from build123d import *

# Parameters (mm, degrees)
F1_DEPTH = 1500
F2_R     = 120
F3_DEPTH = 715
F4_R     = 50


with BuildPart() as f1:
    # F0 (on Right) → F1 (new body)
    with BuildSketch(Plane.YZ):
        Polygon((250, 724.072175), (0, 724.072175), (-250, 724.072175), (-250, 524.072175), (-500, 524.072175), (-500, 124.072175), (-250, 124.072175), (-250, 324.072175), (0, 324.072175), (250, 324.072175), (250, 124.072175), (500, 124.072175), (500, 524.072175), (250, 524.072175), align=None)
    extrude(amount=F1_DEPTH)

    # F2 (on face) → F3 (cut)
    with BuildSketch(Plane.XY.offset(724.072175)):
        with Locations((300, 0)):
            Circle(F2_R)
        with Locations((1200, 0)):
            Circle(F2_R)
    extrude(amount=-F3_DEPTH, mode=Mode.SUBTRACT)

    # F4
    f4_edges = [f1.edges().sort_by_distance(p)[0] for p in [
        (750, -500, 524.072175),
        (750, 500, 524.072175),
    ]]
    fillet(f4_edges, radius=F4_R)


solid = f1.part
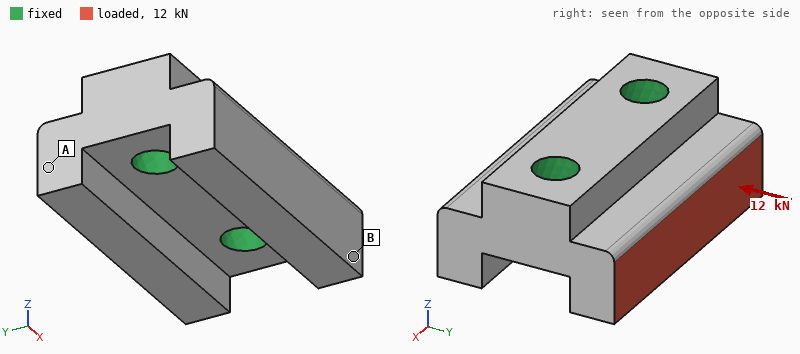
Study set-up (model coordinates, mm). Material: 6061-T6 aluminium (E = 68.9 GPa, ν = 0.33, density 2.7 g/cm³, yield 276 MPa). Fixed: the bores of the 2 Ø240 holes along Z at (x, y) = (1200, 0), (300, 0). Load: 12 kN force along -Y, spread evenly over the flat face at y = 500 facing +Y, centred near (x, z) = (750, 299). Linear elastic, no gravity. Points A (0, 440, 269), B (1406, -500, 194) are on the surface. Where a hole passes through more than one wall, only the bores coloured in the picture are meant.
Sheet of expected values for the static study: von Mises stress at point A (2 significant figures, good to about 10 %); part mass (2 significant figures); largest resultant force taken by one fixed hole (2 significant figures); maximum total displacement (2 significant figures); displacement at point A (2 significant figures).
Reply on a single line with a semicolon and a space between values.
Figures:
0.036 MPa; 1500 kg; 6.0 kN; 2.1 µm; 1.2 µm
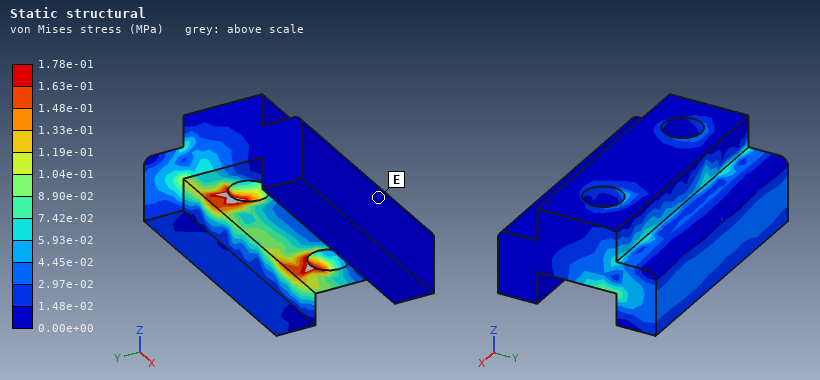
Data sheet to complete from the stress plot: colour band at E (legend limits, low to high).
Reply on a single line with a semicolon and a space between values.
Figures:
0.00e+00 to 1.48e-02 MPa
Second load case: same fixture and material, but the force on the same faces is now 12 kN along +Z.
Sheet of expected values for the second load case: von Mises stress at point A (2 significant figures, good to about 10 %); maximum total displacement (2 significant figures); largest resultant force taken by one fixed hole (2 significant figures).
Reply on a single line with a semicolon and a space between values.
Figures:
0.041 MPa; 4.2 µm; 6.0 kN
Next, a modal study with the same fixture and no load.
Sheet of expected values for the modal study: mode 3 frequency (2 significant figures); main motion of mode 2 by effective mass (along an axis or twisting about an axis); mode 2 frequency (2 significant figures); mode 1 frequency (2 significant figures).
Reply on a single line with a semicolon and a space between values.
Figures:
790 Hz; along Z; 660 Hz; 590 Hz
